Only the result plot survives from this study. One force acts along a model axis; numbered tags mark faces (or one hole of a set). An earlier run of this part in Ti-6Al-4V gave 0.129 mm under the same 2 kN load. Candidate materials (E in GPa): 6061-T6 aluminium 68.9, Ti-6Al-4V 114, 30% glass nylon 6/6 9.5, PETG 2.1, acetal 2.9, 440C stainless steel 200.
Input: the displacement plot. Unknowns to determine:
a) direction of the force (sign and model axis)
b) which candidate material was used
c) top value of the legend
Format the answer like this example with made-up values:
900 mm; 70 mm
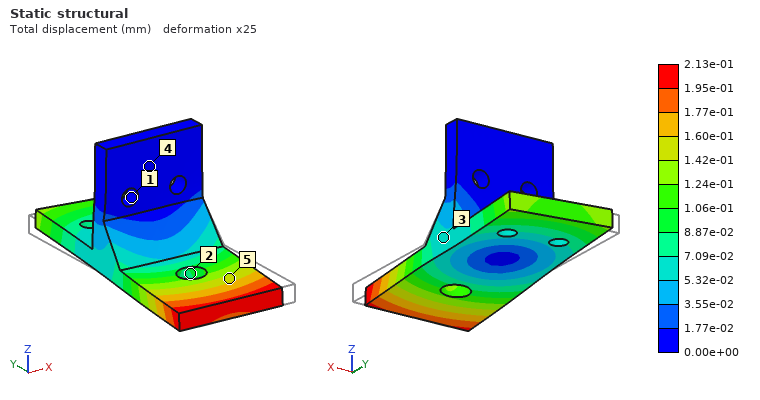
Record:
-X; 6061-T6 aluminium; 2.13e-01 mm
